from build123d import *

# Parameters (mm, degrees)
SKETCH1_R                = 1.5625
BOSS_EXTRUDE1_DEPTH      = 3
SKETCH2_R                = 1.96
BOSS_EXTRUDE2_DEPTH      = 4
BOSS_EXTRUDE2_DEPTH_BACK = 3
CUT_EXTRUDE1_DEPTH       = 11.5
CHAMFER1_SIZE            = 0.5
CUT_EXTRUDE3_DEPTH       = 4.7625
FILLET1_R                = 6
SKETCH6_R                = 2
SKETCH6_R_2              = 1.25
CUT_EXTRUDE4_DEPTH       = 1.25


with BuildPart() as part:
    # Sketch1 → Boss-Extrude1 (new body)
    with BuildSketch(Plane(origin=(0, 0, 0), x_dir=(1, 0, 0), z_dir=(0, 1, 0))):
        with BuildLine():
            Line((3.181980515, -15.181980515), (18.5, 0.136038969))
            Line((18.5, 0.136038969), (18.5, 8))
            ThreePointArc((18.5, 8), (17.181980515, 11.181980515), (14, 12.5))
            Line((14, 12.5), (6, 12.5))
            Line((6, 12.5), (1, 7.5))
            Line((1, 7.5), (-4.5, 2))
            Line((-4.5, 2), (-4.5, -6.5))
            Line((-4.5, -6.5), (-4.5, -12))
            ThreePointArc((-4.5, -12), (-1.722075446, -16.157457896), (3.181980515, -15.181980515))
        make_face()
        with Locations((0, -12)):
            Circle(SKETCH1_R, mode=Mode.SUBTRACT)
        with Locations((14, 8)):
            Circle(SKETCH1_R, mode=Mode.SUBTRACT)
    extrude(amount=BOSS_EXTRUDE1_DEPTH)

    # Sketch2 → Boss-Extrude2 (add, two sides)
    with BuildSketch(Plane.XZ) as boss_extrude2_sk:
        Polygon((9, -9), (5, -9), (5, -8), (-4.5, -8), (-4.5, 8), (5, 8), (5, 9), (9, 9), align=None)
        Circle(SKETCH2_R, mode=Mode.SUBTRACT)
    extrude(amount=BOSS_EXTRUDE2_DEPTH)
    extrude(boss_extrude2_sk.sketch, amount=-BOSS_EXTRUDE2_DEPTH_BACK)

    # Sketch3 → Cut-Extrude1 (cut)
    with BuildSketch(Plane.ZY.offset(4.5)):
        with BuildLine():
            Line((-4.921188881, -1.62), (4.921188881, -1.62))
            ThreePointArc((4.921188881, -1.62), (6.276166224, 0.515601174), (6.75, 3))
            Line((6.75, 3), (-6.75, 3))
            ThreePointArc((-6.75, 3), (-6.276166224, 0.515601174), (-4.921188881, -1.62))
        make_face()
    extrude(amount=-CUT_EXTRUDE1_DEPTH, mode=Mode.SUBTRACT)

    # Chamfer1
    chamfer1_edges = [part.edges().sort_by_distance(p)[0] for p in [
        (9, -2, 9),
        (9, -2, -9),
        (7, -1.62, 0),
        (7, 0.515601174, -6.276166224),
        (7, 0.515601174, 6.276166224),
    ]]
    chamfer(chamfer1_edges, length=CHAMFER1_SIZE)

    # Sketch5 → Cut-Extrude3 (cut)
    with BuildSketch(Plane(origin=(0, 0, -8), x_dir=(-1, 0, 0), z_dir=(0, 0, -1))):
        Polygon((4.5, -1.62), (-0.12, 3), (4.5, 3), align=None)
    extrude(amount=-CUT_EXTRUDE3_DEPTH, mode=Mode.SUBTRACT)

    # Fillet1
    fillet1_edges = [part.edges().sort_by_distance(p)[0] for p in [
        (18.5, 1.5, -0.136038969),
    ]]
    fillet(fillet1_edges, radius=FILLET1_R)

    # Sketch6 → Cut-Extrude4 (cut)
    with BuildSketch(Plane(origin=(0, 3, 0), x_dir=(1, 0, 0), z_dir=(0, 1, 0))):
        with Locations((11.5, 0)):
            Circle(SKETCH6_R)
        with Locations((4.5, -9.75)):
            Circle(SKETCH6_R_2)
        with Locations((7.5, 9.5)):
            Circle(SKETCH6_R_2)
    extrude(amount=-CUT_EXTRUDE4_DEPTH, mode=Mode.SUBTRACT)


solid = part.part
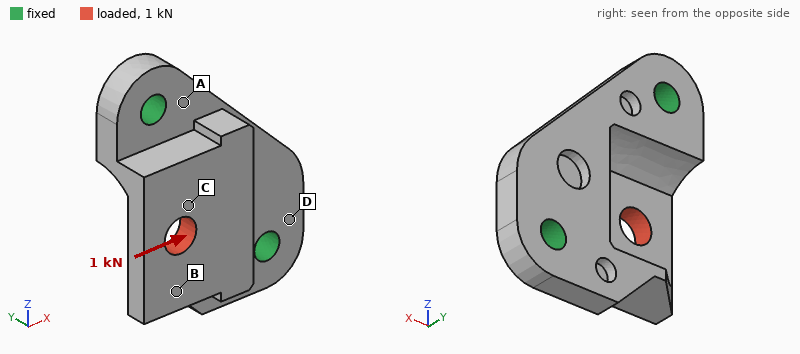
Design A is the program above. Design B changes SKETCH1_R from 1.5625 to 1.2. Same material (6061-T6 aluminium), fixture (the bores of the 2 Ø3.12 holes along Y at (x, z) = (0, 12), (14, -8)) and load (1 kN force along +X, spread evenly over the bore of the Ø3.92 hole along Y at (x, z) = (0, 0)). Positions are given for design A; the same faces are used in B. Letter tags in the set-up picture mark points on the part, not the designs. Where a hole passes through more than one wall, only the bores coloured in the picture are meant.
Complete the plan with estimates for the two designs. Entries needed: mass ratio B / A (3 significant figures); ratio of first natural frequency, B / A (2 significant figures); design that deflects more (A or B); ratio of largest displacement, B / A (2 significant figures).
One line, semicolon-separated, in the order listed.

1.01; 0.93; B; 1.2
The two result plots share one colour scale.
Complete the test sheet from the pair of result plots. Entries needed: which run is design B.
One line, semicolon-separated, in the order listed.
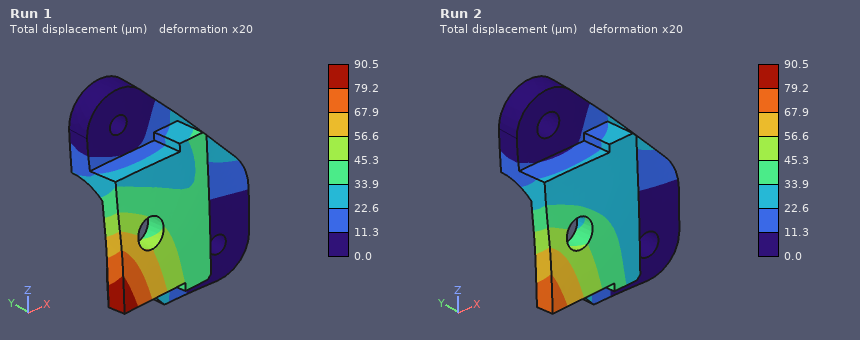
Run 1
